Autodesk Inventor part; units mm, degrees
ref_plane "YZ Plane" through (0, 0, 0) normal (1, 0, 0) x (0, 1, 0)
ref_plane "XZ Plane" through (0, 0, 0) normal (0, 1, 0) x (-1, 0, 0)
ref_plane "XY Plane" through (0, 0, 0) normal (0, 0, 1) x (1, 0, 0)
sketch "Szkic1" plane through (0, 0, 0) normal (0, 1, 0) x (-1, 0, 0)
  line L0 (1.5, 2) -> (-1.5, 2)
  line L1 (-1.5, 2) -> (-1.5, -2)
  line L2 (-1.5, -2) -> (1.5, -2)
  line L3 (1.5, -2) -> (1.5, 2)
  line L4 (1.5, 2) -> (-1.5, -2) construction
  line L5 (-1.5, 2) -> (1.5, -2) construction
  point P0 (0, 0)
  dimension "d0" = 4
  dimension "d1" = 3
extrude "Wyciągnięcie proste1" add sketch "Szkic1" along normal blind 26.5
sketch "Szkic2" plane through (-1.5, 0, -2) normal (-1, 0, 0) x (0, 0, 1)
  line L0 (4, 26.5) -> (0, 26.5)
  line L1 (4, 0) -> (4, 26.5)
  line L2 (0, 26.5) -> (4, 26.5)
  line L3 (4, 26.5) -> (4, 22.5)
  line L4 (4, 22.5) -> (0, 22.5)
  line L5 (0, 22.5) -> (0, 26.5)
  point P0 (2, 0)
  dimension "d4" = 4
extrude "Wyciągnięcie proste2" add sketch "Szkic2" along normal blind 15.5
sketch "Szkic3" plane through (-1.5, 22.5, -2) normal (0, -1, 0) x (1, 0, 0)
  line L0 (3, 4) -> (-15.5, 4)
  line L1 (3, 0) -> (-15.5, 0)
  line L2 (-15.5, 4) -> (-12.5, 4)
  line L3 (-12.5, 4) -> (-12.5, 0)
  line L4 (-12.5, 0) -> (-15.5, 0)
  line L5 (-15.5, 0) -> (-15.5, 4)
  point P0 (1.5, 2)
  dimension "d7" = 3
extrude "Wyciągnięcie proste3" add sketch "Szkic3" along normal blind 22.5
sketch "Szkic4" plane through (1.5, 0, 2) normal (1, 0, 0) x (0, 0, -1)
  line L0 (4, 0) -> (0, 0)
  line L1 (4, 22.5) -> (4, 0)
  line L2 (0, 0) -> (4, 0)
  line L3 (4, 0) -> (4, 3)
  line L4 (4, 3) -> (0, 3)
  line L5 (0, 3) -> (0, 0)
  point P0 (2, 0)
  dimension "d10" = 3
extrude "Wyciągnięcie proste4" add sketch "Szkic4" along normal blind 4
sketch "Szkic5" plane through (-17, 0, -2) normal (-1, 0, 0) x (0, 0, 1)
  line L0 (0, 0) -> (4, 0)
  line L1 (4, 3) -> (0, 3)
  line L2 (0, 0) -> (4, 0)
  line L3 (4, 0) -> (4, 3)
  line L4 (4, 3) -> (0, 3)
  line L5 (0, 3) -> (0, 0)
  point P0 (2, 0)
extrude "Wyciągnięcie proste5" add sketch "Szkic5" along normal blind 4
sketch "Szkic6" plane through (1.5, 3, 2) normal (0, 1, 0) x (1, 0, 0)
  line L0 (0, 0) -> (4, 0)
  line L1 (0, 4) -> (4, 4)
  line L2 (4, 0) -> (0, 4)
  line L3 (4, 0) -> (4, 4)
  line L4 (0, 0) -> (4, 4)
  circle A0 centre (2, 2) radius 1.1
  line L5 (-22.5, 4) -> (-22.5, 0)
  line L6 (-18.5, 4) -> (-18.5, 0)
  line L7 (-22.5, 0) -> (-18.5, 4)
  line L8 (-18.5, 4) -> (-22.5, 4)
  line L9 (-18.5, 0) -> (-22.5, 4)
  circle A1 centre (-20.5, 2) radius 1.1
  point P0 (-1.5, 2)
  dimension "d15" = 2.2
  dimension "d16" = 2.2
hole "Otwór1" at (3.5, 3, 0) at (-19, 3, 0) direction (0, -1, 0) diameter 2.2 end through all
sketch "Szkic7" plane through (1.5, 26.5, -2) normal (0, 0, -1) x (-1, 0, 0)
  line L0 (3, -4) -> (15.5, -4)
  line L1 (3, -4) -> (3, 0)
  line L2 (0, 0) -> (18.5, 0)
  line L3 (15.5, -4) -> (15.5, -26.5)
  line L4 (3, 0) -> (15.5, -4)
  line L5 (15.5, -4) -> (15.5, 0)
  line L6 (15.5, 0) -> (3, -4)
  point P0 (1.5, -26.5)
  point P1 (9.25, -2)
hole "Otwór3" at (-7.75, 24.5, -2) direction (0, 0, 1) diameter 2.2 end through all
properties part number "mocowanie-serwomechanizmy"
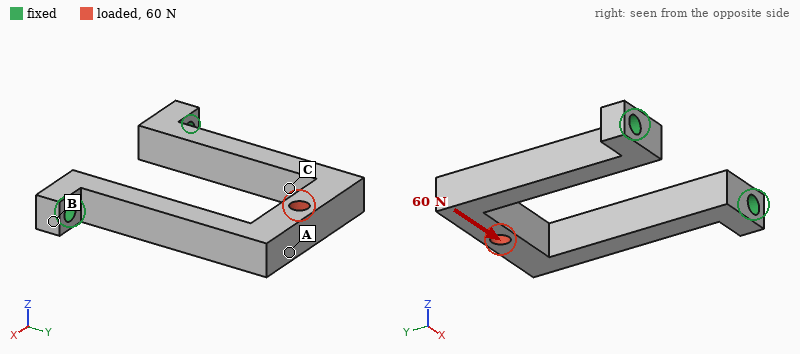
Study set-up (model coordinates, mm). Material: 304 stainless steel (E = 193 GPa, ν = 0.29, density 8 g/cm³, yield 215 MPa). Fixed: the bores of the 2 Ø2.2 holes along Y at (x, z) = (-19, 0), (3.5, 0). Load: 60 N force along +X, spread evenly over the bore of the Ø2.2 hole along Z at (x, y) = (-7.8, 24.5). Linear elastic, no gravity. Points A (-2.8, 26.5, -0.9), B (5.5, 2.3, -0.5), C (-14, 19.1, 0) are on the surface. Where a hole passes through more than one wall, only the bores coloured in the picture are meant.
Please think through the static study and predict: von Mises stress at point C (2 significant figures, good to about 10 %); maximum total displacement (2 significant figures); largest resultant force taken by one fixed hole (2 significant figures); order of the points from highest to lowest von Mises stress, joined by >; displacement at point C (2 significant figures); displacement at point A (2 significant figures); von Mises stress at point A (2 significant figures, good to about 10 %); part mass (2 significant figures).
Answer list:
36 MPa
22 µm
55 N
C > A > B
18 µm
21 µm
20 MPa
7.2 g
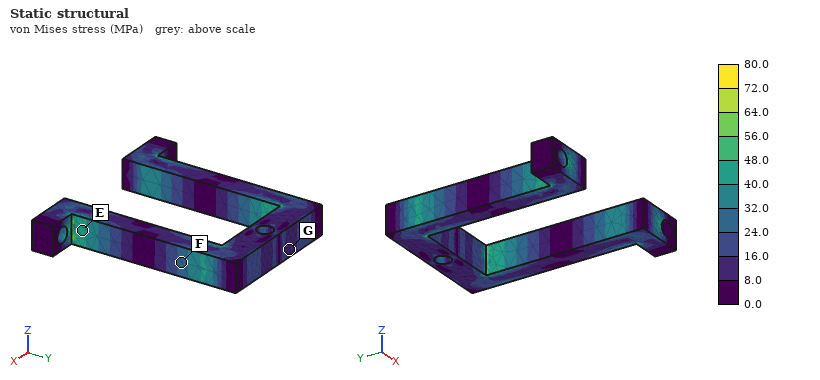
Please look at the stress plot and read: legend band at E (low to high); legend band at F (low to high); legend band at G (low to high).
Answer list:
40.0 to 48.0 MPa
24.0 to 32.0 MPa
8.0 to 16.0 MPa
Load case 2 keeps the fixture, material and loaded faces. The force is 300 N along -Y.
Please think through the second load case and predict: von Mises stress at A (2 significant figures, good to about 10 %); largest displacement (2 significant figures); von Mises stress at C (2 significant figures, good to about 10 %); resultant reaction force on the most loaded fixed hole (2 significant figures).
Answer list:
14 MPa
6.7 µm
40 MPa
150 N
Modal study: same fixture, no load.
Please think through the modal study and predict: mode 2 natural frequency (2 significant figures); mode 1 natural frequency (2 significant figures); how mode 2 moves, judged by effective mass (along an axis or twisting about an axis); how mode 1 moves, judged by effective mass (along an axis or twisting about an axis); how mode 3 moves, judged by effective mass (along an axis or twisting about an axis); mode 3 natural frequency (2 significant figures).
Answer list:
4500 Hz
2900 Hz
along X
along Z
twisting about Y
7000 Hz
